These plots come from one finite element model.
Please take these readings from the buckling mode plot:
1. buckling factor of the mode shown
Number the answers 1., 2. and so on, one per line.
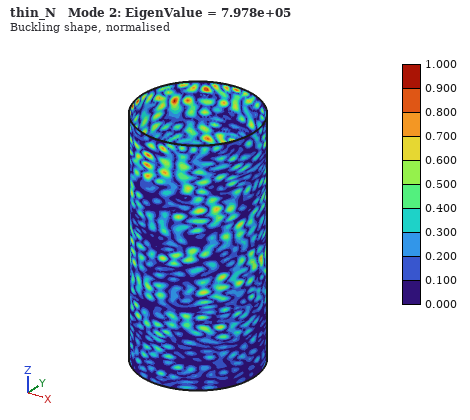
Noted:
1. 7.978e+05
